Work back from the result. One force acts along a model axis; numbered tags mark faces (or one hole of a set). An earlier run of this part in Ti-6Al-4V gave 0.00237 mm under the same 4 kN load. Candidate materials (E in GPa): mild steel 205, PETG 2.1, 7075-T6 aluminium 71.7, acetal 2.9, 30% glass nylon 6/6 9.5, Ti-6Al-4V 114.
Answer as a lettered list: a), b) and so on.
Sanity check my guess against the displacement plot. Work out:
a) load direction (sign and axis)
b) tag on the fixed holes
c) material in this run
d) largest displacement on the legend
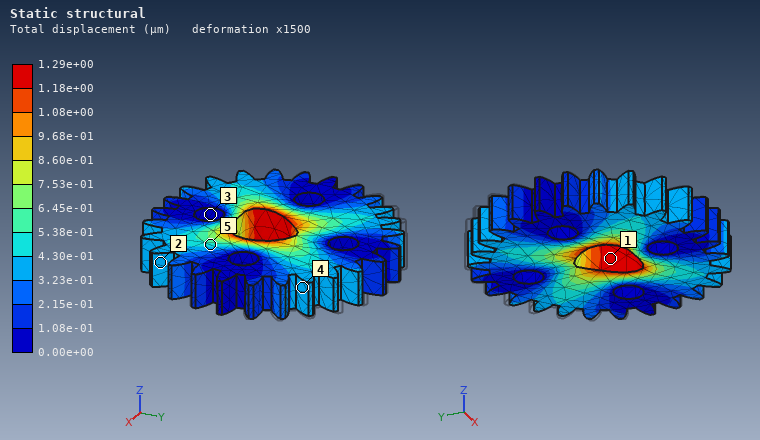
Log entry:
a) -Y
b) 3
c) mild steel
d) 1.29e+00 µm
